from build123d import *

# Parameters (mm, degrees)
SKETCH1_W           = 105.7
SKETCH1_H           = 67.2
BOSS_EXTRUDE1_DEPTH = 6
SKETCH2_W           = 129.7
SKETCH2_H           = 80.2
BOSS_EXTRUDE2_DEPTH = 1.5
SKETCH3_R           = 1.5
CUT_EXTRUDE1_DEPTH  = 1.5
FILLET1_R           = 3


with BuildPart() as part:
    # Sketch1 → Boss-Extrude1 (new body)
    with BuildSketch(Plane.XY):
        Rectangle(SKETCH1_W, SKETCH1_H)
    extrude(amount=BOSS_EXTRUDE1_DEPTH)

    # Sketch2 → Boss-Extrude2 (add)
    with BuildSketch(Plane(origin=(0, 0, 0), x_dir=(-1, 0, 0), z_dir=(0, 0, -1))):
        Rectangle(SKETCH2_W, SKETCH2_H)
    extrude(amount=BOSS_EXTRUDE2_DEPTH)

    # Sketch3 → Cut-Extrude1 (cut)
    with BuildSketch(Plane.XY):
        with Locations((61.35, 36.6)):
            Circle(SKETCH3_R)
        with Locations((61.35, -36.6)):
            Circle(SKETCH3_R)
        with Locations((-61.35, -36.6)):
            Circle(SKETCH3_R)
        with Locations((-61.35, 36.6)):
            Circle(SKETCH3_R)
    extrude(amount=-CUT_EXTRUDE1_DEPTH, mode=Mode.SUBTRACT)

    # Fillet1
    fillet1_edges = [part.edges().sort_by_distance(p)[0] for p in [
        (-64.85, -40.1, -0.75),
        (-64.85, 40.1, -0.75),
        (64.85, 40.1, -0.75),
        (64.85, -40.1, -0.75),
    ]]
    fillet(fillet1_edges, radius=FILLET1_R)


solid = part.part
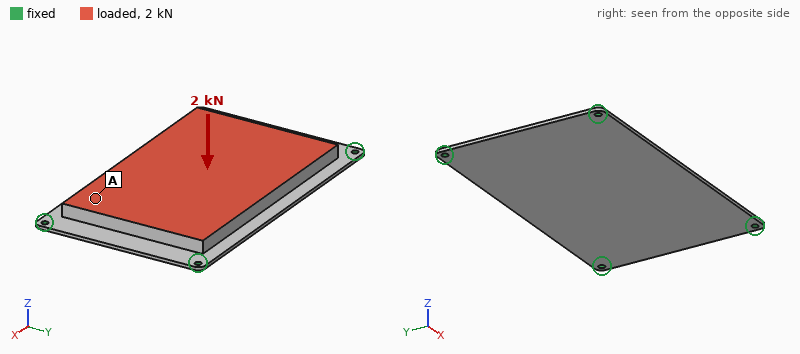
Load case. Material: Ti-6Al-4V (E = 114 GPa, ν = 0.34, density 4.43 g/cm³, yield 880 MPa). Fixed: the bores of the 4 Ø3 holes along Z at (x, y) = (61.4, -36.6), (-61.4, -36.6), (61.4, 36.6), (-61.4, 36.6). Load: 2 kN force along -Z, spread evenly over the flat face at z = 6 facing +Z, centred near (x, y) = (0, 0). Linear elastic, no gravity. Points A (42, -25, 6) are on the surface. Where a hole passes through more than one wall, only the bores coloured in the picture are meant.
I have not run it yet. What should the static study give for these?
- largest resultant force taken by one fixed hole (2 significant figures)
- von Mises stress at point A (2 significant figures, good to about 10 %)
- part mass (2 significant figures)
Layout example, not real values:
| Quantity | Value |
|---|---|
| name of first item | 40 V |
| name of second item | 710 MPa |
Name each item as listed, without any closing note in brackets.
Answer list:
| Quantity | Value |
|---|---|
| largest resultant force taken by one fixed hole | 1.2 kN |
| von Mises stress at point A | 33 MPa |
| part mass | 260 g |
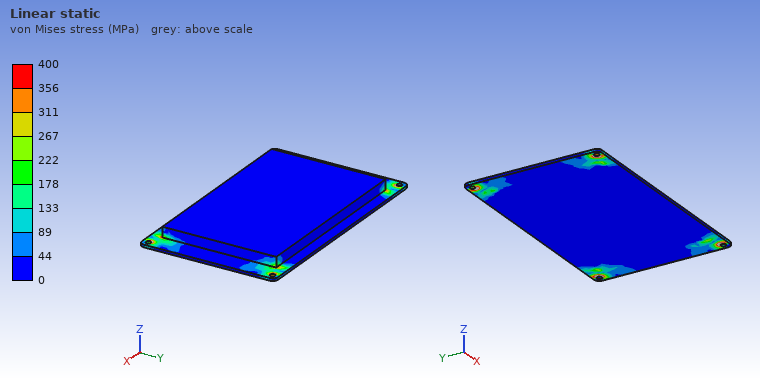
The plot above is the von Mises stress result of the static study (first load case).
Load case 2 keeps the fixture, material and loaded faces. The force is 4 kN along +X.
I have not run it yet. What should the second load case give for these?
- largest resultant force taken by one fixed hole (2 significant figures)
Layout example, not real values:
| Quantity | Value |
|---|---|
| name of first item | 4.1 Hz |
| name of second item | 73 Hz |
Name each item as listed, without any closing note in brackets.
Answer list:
| Quantity | Value |
|---|---|
| largest resultant force taken by one fixed hole | 1.1 kN |
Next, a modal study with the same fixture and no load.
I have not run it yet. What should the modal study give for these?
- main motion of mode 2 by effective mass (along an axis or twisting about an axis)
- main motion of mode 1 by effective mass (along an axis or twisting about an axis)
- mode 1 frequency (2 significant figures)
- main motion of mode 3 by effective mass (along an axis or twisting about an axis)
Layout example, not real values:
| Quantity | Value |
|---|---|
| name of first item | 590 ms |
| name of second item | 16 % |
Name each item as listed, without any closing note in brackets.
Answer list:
| Quantity | Value |
|---|---|
| main motion of mode 2 by effective mass | twisting about X |
| main motion of mode 1 by effective mass | along Z |
| mode 1 frequency | 1000 Hz |
| main motion of mode 3 by effective mass | twisting about Y |
